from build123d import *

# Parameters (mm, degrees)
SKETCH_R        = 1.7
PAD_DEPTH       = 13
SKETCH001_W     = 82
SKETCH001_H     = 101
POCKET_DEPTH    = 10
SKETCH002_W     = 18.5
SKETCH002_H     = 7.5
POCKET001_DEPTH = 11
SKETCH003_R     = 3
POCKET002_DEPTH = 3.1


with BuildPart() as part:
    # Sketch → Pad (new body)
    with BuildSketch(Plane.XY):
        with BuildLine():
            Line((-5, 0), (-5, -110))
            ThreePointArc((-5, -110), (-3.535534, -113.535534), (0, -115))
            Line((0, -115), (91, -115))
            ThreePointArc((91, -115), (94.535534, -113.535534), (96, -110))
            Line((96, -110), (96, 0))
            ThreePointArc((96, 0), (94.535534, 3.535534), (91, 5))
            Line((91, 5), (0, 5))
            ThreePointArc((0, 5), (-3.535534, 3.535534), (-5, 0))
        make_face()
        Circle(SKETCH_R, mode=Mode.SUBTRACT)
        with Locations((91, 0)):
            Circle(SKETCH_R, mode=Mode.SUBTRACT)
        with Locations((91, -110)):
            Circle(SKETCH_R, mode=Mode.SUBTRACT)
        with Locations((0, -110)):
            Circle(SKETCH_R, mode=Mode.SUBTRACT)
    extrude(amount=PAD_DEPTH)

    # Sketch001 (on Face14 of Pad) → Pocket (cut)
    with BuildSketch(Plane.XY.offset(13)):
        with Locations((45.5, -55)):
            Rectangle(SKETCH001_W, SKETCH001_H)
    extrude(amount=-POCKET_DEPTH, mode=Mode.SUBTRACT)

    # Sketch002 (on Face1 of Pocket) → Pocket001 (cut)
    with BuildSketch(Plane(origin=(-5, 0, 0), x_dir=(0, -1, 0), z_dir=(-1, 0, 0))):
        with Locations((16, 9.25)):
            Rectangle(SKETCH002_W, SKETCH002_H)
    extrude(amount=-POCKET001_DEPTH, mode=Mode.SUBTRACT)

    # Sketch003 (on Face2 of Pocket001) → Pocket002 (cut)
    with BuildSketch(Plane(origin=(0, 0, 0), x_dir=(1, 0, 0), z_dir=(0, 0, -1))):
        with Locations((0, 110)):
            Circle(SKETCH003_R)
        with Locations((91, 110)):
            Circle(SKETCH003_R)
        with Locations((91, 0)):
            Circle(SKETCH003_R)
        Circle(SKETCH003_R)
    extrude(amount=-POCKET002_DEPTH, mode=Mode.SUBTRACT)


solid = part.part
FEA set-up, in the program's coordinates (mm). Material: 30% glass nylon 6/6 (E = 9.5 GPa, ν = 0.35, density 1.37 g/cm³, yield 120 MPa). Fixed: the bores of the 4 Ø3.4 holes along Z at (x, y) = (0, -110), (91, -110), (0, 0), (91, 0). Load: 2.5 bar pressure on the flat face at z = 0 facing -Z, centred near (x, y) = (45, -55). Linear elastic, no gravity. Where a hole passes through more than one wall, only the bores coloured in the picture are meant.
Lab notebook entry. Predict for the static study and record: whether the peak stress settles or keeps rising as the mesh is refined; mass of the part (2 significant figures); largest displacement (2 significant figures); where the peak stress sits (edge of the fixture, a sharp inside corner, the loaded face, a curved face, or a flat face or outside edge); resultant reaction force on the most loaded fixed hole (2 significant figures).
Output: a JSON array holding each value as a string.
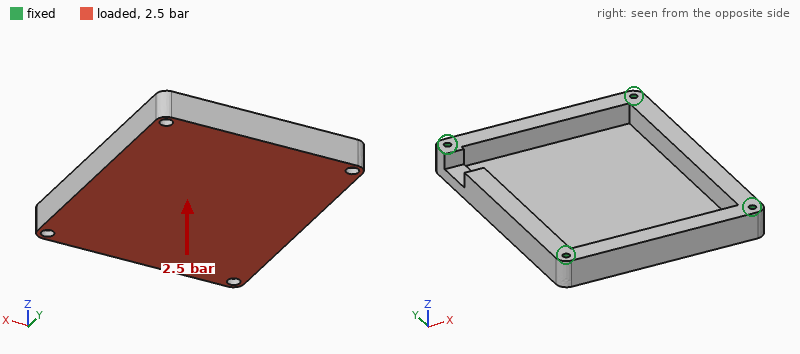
["keeps rising", "99 g", "1.6 mm", "edge of the fixture", "1.2 kN"]
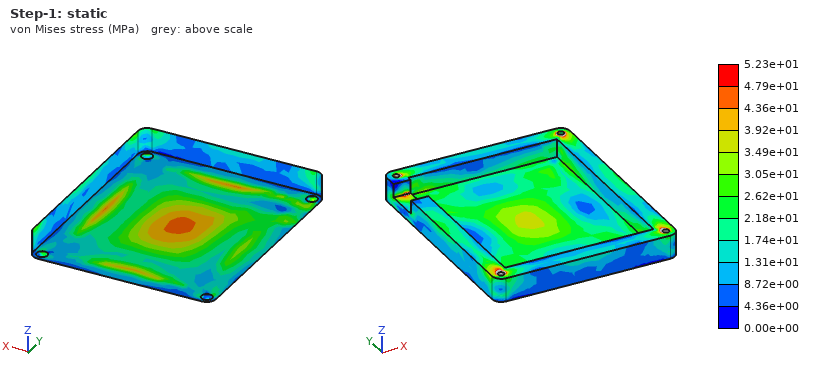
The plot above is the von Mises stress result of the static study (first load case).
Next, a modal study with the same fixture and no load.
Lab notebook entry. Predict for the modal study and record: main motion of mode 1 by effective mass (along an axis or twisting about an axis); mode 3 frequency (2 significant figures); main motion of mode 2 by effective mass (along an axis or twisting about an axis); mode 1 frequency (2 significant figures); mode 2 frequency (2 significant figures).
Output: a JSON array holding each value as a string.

["along Z", "2300 Hz", "twisting about Y", "1200 Hz", "1900 Hz"]
